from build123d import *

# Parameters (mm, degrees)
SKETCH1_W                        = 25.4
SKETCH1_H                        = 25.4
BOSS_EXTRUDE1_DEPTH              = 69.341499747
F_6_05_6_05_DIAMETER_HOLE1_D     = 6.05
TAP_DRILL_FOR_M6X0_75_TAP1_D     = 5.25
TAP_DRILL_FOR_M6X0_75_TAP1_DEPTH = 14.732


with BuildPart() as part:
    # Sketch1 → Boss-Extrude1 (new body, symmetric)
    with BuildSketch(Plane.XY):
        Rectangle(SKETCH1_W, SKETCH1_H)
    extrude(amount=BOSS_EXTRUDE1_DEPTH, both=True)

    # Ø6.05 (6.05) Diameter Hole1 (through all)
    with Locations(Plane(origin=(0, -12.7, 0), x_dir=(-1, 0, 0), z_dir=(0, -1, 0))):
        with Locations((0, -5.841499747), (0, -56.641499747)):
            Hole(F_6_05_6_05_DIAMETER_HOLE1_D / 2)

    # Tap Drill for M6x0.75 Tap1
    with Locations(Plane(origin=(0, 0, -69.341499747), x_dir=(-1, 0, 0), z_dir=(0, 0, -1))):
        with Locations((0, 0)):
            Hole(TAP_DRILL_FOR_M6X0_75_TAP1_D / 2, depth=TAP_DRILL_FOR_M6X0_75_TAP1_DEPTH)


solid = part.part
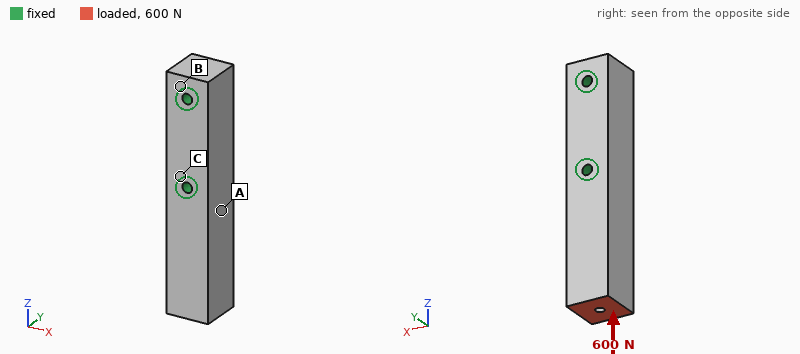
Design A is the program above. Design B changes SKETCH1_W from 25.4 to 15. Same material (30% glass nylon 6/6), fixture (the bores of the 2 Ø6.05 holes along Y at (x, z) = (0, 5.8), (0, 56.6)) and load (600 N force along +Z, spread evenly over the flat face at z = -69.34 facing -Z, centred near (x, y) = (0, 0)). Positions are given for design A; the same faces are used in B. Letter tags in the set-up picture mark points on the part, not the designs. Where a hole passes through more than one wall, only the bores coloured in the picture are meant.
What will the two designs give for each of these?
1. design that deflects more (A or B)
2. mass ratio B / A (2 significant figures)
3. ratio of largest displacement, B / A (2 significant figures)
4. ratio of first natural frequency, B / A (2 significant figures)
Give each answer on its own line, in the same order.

B
0.58
1.6
0.73
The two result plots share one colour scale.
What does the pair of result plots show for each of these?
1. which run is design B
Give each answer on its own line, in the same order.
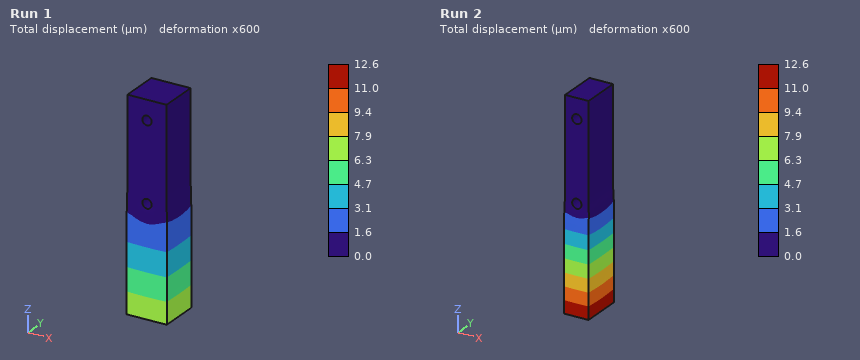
Run 2
